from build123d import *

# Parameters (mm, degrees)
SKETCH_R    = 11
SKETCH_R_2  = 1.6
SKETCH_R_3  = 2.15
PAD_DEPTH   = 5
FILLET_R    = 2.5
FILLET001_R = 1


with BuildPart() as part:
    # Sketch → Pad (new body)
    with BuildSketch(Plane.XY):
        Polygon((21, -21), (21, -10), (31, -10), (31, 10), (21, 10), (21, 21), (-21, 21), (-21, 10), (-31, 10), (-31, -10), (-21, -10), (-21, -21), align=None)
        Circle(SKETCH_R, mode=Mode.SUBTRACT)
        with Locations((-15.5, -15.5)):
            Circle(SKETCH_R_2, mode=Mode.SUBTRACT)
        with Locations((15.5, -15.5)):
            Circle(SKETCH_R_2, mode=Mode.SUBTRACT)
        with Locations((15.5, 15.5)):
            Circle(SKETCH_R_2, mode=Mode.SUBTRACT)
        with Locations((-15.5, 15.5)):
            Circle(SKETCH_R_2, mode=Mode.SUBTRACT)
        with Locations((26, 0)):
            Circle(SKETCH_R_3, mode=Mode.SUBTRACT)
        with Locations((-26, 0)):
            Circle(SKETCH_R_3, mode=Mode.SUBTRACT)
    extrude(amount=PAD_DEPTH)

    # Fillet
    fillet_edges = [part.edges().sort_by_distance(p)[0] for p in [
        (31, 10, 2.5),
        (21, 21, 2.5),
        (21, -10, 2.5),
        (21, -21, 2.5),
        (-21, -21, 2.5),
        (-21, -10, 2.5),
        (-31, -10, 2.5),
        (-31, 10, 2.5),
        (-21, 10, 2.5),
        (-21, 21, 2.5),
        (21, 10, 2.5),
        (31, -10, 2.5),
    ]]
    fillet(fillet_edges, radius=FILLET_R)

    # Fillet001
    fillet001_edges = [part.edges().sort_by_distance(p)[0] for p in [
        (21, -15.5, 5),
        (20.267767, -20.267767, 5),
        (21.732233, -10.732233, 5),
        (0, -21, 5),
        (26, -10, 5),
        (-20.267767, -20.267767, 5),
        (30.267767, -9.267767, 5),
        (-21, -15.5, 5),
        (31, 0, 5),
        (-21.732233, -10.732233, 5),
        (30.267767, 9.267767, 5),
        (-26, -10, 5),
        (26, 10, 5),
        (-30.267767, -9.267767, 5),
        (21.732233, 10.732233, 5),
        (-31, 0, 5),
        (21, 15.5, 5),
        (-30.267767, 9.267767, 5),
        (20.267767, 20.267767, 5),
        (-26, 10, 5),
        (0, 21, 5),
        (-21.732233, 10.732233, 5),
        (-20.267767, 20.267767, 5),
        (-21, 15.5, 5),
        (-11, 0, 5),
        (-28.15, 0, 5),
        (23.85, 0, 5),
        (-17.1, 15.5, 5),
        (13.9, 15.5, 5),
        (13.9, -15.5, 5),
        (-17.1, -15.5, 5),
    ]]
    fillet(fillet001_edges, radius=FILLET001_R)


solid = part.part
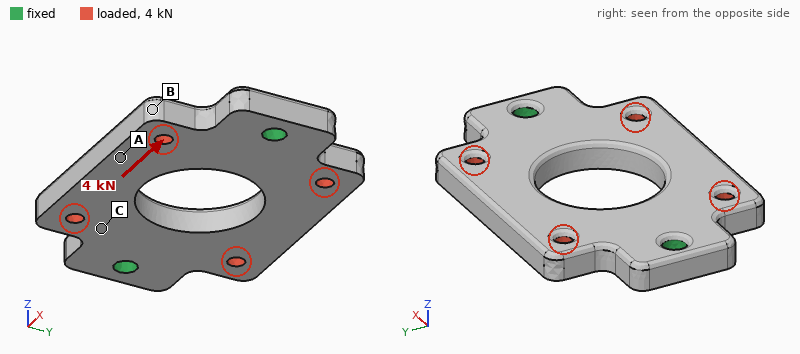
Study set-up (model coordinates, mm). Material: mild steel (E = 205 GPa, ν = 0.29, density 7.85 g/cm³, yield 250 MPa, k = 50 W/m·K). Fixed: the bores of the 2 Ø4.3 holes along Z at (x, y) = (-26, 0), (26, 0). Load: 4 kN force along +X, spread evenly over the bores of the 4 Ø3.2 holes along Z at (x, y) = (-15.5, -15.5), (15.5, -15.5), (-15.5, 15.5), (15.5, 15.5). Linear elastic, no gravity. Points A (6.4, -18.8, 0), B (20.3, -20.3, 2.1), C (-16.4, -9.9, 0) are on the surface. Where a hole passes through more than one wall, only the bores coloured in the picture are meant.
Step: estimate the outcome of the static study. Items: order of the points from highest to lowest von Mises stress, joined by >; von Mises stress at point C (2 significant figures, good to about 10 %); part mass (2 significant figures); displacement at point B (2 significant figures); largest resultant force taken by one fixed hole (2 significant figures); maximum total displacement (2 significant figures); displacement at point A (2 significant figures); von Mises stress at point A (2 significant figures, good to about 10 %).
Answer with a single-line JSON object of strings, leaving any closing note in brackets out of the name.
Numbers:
{"order of the points from highest to lowest von Mises stress, joined by >": "C > A > B", "von Mises stress at point C": "29 MPa", "part mass": "67 g", "displacement at point B": "4.2 µm", "largest resultant force taken by one fixed hole": "2.0 kN", "maximum total displacement": "4.4 µm", "displacement at point A": "3.4 µm", "von Mises stress at point A": "15 MPa"}
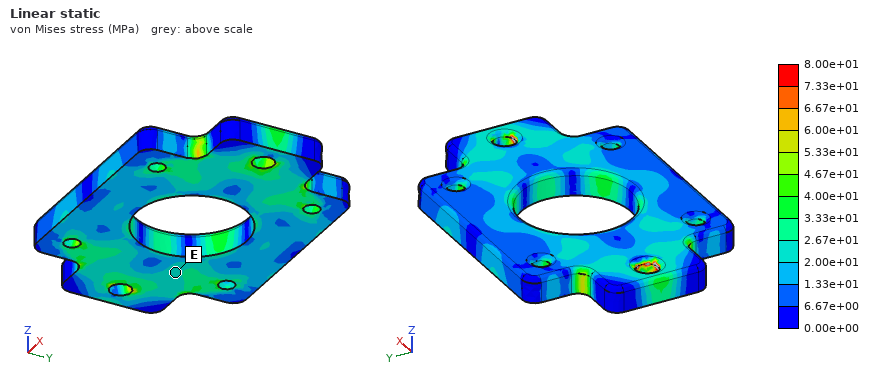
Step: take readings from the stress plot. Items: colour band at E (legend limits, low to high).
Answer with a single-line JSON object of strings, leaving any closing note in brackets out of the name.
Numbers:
{"colour band at E": "2.00e+01 to 2.67e+01 MPa"}
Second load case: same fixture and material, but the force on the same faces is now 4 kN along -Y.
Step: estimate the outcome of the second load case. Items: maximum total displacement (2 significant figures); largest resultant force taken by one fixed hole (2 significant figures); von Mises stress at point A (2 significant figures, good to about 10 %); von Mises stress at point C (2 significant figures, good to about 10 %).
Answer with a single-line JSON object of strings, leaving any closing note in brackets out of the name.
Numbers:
{"maximum total displacement": "6.3 µm", "largest resultant force taken by one fixed hole": "2.0 kN", "von Mises stress at point A": "7.2 MPa", "von Mises stress at point C": "26 MPa"}
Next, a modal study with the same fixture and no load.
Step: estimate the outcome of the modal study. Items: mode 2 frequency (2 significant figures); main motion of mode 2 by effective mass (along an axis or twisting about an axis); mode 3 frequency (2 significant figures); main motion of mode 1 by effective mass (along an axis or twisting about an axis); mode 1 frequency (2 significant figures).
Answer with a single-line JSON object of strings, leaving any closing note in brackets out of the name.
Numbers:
{"mode 2 frequency": "6100 Hz", "main motion of mode 2 by effective mass": "along Z", "mode 3 frequency": "12 kHz", "main motion of mode 1 by effective mass": "twisting about X", "mode 1 frequency": "5100 Hz"}
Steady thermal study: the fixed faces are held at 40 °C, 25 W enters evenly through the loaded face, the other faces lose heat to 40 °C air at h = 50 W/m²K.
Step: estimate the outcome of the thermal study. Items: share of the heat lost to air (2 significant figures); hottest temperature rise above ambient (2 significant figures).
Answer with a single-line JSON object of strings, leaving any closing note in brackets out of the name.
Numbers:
{"share of the heat lost to air": "21 %", "hottest temperature rise above ambient": "38 K"}
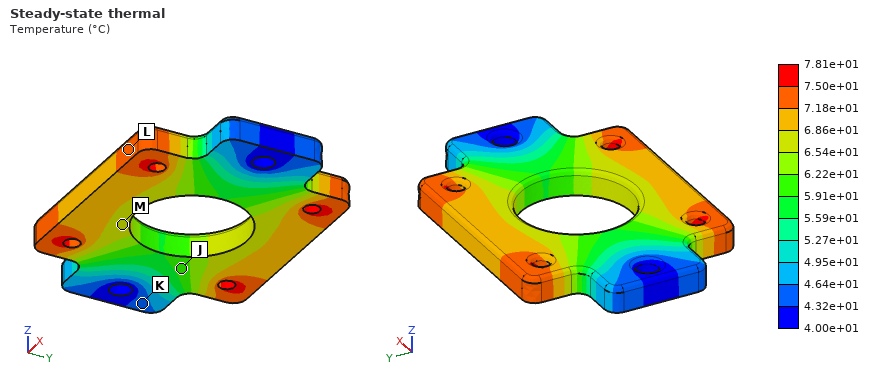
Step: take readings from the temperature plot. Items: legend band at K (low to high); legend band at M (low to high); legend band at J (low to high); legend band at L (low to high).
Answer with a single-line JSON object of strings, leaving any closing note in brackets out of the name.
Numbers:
{"legend band at K": "4.32e+01 to 4.64e+01 °C", "legend band at M": "6.54e+01 to 6.86e+01 °C", "legend band at J": "5.91e+01 to 6.22e+01 °C", "legend band at L": "7.18e+01 to 7.50e+01 °C"}
